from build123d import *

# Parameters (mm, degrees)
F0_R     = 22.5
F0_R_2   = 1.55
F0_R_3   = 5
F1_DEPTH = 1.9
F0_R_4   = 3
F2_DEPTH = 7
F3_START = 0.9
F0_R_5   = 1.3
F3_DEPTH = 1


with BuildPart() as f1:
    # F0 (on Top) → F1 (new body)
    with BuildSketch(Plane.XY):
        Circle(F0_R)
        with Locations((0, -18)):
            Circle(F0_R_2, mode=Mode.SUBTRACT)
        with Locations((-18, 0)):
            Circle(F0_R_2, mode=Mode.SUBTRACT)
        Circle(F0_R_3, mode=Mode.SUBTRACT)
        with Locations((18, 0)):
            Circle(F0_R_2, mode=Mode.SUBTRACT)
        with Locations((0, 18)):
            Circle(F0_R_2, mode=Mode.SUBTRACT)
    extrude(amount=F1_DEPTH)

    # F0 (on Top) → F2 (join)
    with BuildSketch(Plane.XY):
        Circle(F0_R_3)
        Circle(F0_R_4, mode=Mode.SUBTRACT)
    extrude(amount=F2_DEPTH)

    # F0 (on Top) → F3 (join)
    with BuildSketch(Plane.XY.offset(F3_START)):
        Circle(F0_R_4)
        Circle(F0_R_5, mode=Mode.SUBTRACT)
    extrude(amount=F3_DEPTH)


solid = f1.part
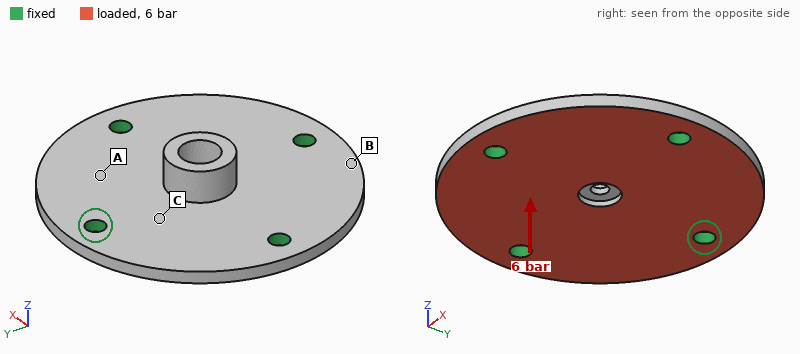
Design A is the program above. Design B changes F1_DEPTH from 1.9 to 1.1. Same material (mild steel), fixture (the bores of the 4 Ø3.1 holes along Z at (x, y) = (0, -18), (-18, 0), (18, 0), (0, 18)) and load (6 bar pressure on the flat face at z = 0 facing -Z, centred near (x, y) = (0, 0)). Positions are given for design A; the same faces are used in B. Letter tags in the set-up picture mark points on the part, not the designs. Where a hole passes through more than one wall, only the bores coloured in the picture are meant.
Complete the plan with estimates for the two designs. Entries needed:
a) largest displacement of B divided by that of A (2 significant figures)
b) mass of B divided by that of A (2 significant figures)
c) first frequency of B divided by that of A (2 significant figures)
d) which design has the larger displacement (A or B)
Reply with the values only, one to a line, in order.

4.9
0.63
0.55
B
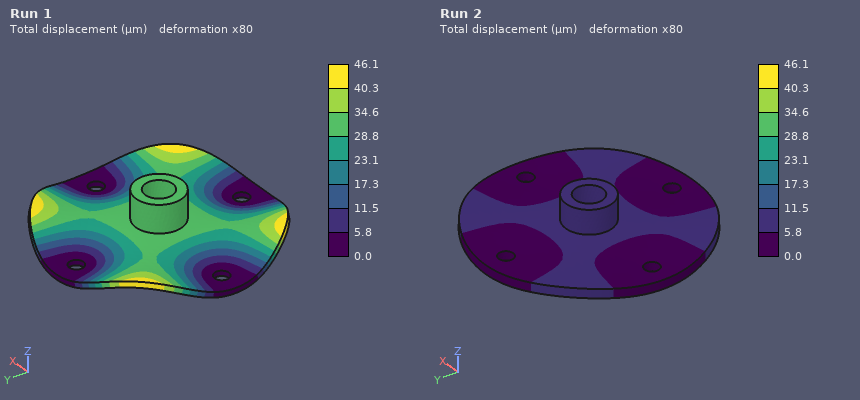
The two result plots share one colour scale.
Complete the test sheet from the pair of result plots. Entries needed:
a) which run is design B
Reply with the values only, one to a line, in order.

Run 1
